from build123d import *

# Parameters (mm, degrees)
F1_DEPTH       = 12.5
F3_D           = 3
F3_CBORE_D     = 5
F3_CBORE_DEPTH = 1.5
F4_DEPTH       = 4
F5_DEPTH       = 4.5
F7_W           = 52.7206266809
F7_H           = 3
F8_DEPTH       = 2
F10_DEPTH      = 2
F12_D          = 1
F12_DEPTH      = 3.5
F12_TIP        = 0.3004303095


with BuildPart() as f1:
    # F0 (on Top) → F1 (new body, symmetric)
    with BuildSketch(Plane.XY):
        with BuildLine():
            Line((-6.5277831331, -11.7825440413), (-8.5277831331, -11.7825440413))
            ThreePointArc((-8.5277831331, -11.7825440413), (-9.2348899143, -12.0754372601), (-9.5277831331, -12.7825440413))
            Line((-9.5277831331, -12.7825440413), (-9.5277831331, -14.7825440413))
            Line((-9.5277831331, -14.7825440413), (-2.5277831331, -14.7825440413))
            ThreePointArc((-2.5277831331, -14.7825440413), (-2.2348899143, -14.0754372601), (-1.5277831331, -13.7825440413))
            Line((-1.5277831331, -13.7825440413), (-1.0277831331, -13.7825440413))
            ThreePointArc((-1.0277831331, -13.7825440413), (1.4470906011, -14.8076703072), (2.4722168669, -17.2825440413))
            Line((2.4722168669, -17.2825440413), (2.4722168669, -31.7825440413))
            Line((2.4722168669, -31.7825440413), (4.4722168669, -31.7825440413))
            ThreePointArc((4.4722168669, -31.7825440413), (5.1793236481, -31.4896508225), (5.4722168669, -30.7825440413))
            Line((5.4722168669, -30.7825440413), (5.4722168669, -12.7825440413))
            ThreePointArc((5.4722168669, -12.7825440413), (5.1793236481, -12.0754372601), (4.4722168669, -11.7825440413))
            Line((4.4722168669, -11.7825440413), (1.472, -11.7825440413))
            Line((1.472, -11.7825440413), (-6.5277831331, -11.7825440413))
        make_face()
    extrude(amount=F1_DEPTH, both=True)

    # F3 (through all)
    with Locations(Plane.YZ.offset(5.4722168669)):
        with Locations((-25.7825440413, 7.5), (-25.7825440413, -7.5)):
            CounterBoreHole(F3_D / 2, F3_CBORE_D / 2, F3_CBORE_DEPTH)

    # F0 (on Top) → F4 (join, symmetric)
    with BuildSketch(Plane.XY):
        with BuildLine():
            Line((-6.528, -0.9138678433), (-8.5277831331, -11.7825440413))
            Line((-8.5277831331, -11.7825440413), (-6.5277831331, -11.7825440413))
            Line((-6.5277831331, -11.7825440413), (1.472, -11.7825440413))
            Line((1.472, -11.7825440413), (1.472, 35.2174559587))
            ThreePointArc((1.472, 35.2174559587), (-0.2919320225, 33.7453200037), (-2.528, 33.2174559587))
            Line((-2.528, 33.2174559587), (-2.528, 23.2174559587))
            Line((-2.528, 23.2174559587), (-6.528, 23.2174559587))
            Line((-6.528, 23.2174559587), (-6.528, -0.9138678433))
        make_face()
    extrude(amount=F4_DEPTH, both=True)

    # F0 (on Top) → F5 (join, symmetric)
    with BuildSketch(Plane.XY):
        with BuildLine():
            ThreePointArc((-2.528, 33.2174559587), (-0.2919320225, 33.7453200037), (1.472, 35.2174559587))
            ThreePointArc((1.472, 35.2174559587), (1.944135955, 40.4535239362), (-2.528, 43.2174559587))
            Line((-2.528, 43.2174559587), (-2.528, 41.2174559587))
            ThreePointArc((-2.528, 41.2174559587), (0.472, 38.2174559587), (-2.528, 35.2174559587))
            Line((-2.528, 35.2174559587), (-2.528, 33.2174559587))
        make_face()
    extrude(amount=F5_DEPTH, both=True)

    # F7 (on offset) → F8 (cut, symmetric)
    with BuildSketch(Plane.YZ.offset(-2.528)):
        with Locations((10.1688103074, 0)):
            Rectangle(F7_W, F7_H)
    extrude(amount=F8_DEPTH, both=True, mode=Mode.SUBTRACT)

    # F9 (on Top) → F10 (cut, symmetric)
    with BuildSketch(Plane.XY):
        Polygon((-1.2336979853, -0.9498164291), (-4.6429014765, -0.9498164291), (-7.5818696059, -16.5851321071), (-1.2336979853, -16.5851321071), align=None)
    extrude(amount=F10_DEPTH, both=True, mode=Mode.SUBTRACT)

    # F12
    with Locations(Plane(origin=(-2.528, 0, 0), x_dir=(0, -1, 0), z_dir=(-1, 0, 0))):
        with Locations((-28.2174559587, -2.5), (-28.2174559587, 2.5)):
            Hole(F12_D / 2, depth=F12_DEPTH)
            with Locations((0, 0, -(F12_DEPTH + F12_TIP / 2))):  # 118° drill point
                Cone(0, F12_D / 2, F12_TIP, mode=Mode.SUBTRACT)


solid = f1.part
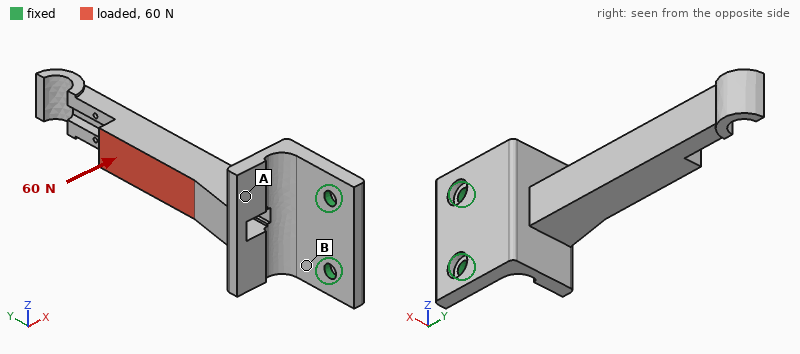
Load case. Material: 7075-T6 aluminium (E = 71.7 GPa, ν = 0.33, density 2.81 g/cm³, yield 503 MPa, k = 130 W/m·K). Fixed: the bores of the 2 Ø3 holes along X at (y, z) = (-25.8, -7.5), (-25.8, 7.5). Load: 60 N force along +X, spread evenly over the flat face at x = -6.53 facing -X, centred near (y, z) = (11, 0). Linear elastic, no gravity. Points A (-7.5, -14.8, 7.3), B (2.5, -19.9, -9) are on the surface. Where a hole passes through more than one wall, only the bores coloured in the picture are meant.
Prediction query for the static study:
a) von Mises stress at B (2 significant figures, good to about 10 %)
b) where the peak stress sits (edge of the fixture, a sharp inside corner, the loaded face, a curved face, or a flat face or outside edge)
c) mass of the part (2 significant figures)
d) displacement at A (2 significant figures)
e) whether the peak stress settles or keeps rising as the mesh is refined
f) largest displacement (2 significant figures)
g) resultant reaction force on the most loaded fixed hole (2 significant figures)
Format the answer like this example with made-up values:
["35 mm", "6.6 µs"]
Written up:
["45 MPa", "edge of the fixture", "13 g", "0.11 mm", "keeps rising", "0.64 mm", "40 N"]
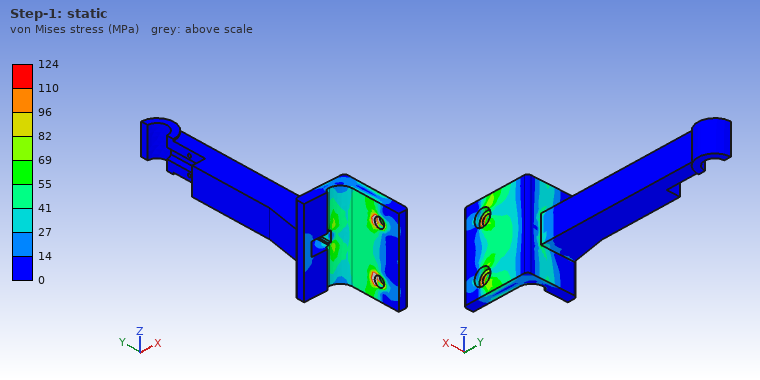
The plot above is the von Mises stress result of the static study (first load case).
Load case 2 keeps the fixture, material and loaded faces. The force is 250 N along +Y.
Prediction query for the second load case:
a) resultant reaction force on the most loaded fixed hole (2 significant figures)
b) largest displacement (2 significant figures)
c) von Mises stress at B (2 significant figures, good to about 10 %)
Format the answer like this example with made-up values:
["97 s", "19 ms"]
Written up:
["140 N", "0.82 mm", "66 MPa"]
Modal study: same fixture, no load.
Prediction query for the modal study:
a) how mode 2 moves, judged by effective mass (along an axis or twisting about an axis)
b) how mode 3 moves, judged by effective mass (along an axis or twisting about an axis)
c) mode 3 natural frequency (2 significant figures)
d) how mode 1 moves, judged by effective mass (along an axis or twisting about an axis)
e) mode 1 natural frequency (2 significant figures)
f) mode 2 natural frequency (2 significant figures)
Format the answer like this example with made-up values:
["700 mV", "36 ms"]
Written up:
["along Z", "along X", "5300 Hz", "along X", "750 Hz", "2100 Hz"]
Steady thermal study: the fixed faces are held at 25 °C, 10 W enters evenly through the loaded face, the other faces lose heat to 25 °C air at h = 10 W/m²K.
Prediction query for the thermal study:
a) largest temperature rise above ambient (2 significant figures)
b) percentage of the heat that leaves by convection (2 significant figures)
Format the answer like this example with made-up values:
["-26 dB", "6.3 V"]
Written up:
["52 K", "11 %"]
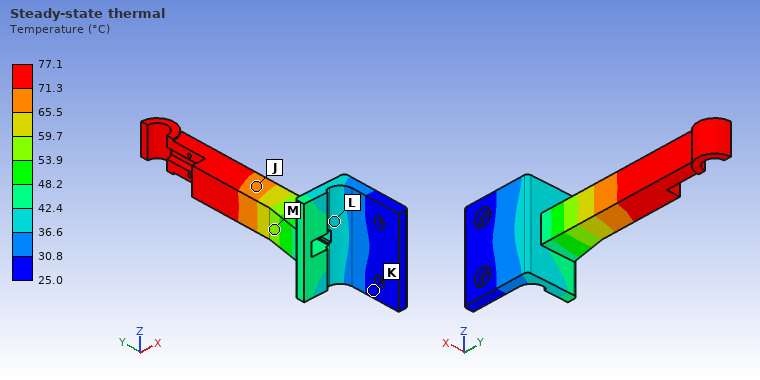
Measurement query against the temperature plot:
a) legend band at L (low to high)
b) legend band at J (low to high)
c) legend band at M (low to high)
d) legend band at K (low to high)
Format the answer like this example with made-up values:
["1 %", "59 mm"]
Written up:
["36.6 to 42.4 °C", "65.5 to 71.3 °C", "53.9 to 59.7 °C", "25.0 to 30.8 °C"]
